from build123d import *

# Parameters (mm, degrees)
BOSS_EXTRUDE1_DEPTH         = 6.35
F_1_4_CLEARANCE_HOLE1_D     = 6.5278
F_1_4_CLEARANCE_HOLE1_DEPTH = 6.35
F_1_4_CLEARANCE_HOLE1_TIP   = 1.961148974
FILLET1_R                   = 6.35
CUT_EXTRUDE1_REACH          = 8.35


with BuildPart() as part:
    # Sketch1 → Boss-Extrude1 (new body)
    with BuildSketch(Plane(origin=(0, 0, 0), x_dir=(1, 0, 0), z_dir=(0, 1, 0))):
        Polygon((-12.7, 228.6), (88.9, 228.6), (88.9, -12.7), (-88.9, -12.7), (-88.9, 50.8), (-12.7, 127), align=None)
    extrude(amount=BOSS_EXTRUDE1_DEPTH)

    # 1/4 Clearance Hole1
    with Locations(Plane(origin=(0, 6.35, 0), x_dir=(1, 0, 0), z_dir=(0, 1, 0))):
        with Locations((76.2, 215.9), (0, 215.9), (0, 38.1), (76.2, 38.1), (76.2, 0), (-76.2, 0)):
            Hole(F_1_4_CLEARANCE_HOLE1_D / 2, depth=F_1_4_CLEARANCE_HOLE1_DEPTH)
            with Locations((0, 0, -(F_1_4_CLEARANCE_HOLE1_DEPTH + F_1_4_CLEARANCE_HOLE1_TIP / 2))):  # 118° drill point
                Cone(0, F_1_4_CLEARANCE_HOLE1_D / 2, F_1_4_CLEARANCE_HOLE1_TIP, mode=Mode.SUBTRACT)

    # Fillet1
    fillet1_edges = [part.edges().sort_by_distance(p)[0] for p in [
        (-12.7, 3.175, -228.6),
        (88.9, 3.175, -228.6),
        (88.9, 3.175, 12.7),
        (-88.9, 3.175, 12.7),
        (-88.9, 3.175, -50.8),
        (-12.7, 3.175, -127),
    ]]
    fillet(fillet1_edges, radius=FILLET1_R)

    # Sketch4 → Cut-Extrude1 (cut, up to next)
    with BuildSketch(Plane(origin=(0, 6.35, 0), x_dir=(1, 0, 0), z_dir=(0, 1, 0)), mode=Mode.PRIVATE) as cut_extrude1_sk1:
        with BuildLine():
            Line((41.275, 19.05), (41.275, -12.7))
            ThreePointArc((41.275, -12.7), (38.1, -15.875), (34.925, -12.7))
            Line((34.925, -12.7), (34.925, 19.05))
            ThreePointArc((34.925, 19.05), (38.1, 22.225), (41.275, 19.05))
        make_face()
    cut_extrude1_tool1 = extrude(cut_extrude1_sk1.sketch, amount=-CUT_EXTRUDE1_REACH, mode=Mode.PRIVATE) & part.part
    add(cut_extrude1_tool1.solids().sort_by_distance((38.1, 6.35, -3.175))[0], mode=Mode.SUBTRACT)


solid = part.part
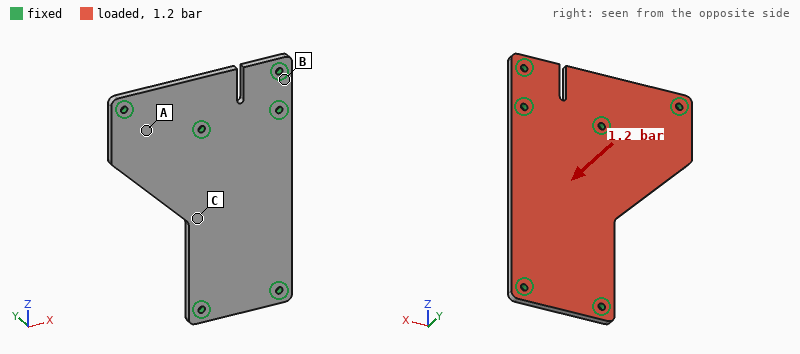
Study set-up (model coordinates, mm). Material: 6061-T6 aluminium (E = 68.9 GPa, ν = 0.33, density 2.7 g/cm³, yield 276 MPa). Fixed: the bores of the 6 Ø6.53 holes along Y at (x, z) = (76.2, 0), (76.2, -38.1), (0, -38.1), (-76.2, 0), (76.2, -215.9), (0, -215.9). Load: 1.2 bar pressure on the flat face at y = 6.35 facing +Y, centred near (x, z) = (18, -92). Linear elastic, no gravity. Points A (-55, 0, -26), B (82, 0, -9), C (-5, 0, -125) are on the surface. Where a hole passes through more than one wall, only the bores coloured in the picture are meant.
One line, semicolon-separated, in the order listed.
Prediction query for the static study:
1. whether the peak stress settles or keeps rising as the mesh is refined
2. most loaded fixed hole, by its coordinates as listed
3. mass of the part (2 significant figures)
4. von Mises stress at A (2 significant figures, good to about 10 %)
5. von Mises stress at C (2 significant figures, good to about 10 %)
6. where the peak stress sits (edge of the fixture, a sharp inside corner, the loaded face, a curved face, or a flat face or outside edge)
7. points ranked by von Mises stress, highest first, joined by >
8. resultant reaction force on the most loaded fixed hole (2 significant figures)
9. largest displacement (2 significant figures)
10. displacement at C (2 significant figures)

keeps rising; (0, -38.1); 550 g; 15 MPa; 30 MPa; edge of the fixture; C > A > B; 1.4 kN; 0.28 mm; 0.27 mm
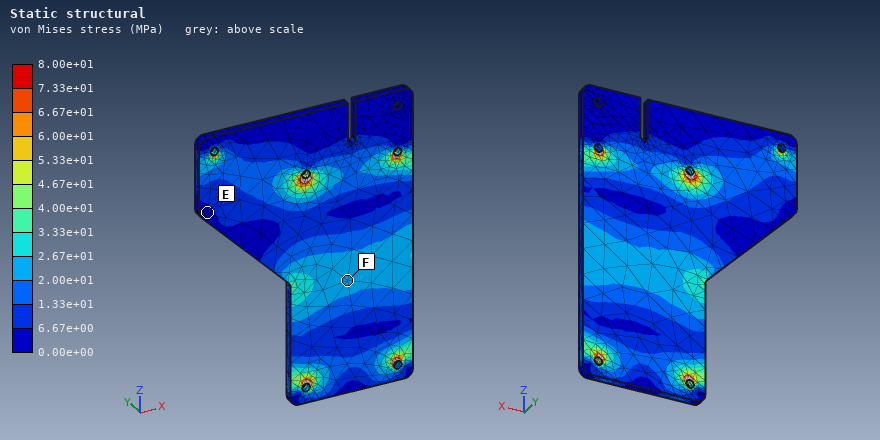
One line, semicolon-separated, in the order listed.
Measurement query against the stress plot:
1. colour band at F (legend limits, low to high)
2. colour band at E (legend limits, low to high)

2.00e+01 to 2.67e+01 MPa; 0.00e+00 to 6.67e+00 MPa
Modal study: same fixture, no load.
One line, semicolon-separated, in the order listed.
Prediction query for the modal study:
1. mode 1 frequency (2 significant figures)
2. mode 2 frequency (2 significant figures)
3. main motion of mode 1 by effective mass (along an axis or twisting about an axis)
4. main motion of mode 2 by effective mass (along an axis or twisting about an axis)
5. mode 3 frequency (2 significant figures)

950 Hz; 1300 Hz; along Y; twisting about Z; 2000 Hz
